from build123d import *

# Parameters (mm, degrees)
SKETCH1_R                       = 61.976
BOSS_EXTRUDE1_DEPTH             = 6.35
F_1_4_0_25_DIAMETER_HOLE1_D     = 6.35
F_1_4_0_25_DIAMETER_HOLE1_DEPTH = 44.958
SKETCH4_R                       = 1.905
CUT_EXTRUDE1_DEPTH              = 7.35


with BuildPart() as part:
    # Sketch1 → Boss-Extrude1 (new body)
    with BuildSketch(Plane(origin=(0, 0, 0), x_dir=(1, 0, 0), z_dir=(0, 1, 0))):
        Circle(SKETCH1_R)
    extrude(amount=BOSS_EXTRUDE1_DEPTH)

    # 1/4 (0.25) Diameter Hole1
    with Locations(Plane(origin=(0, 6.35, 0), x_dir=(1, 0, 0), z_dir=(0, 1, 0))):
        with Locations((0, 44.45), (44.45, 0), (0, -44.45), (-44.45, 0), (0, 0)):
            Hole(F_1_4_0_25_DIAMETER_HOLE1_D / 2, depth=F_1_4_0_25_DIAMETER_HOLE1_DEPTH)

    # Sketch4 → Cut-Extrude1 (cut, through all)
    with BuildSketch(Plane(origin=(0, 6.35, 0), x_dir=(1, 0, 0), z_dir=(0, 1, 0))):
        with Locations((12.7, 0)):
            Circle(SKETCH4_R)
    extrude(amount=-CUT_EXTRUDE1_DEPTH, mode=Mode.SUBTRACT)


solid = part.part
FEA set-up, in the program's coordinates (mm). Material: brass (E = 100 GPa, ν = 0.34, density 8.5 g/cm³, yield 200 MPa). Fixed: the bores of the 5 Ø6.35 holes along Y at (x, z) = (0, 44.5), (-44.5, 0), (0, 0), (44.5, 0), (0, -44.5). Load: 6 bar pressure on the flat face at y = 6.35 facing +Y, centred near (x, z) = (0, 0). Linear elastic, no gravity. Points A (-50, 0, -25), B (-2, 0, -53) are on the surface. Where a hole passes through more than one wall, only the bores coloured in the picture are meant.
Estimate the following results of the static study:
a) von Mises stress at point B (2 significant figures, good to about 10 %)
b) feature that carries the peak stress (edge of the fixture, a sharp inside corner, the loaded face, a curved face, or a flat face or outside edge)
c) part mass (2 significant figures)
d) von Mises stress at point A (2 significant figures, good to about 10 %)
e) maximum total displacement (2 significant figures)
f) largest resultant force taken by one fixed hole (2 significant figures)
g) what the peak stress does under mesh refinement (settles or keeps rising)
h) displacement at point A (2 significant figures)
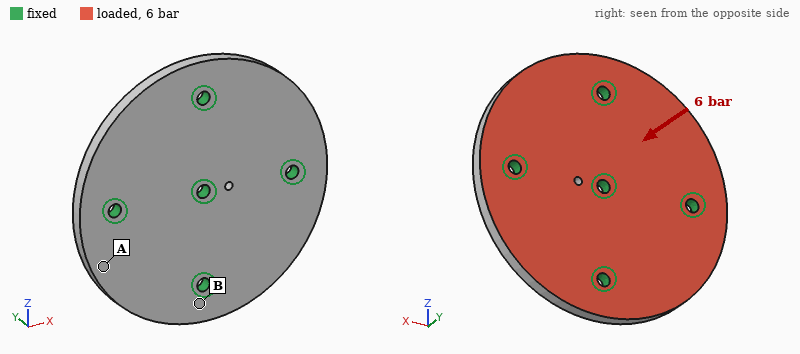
27 MPa
edge of the fixture
640 g
7.7 MPa
38 µm
1.5 kN
keeps rising
22 µm
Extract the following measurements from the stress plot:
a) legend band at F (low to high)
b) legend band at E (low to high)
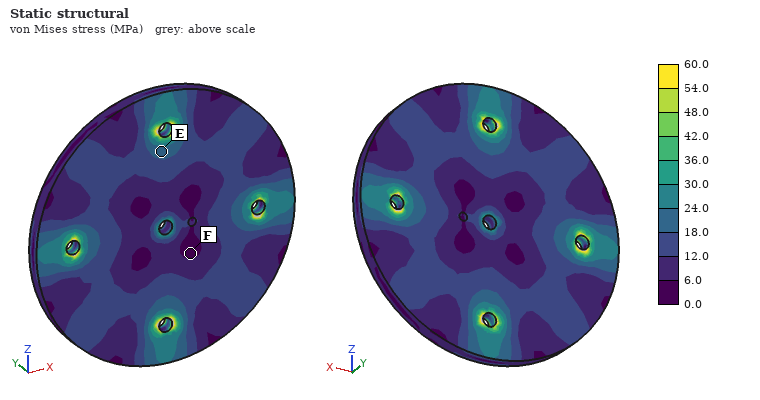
0.0 to 6.0 MPa
18.0 to 24.0 MPa
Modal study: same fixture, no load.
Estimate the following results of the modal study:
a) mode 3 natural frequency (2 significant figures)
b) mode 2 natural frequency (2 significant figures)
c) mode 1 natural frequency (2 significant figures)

3400 Hz
3400 Hz
3100 Hz
